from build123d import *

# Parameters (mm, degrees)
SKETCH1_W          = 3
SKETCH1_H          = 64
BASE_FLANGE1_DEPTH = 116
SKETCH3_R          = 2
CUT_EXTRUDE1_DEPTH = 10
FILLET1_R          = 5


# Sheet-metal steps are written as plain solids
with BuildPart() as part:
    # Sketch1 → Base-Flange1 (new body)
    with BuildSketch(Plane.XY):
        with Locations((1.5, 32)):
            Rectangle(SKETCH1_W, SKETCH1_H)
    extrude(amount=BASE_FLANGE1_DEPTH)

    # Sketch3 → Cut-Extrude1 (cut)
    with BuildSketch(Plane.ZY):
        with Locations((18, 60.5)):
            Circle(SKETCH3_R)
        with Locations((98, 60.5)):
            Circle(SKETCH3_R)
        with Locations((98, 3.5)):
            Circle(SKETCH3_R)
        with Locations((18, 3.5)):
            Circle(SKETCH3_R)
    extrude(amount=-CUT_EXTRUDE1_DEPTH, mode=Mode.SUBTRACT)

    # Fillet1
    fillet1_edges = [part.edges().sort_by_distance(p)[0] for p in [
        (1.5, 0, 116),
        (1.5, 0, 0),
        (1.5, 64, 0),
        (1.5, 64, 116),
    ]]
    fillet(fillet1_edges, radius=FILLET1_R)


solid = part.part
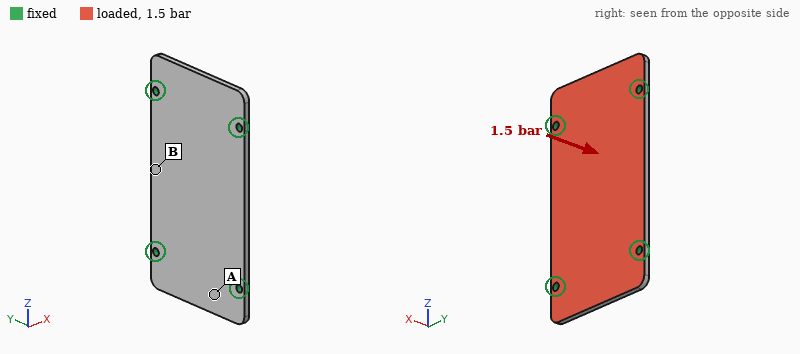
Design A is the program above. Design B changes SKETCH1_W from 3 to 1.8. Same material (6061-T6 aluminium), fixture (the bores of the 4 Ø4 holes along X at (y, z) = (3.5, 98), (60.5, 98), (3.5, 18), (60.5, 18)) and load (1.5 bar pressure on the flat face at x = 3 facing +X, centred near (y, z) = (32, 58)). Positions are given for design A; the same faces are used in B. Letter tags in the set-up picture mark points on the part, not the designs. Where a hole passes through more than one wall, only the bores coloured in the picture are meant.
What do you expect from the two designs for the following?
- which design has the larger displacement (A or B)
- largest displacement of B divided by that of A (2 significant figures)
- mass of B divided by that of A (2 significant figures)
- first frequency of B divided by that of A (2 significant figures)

B
4.4
0.60
0.62
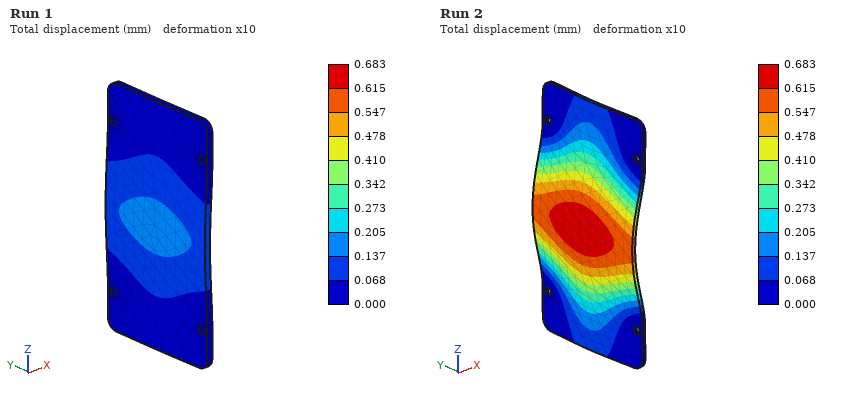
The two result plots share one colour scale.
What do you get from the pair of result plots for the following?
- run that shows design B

Run 2
